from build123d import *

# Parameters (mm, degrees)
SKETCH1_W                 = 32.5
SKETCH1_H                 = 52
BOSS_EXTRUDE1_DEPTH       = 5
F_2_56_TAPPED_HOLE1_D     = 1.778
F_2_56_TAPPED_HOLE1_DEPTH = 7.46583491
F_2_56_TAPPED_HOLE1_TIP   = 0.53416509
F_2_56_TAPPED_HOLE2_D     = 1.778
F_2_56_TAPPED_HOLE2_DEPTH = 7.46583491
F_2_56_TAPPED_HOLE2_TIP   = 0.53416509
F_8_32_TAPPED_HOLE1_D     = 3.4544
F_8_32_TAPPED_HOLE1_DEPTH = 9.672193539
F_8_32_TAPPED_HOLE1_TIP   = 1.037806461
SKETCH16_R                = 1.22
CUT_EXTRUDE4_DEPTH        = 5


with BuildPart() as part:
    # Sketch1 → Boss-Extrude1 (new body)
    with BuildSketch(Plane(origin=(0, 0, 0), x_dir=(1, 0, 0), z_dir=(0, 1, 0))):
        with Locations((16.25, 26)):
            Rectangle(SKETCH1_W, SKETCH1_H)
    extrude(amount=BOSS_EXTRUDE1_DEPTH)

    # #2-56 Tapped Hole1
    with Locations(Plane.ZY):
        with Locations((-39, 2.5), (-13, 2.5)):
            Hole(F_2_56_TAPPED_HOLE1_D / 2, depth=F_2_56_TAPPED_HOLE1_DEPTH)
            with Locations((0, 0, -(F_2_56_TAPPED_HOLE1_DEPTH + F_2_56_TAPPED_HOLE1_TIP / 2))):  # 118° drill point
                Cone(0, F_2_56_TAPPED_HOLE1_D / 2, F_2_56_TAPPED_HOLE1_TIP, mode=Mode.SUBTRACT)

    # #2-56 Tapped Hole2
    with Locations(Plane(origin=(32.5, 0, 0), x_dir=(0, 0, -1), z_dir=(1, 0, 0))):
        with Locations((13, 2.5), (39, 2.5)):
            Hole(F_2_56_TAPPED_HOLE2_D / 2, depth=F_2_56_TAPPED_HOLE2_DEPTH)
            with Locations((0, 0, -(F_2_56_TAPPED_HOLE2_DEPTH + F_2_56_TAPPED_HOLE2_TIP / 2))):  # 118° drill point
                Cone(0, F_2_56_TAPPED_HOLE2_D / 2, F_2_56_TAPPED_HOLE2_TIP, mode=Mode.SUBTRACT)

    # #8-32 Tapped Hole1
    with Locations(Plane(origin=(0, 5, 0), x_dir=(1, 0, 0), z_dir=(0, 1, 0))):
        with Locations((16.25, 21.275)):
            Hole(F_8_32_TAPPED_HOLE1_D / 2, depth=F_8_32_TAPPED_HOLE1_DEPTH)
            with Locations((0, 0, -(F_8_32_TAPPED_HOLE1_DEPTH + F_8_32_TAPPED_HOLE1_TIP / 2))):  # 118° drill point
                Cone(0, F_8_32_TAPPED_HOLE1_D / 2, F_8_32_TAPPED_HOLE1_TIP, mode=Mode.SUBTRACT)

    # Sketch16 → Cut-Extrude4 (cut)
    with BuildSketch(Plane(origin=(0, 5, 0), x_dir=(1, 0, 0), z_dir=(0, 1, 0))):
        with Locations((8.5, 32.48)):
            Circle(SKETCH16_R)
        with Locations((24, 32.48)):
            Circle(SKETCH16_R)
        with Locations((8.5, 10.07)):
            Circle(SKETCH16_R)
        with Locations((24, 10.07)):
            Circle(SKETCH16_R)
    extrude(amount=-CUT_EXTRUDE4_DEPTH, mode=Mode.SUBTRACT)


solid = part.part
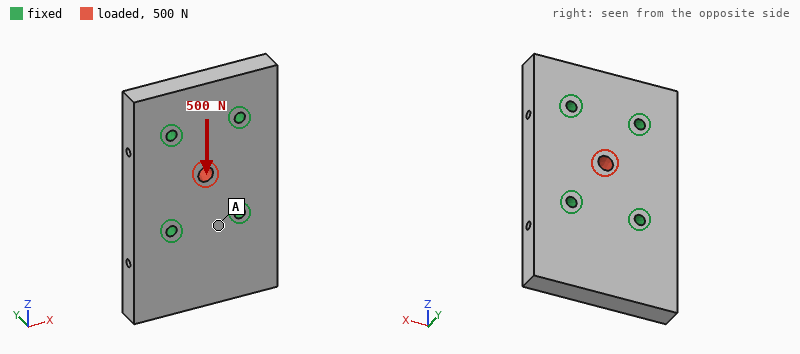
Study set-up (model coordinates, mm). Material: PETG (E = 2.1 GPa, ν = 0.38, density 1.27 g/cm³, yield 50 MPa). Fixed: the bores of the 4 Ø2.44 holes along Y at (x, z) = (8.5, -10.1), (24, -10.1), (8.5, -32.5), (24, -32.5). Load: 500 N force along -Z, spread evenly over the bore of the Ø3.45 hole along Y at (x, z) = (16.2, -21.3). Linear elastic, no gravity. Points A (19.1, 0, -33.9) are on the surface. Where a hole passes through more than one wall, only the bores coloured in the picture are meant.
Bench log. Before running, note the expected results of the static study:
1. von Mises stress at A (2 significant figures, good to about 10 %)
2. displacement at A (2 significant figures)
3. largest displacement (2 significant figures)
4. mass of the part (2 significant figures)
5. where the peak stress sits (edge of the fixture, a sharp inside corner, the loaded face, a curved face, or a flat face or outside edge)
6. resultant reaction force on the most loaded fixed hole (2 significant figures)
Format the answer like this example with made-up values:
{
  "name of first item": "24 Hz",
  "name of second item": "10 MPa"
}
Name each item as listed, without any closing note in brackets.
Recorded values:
{
  "von Mises stress at A": "1.5 MPa",
  "displacement at A": "7.1 µm",
  "largest displacement": "30 µm",
  "mass of the part": "10 g",
  "where the peak stress sits": "the loaded face",
  "resultant reaction force on the most loaded fixed hole": "130 N"
}
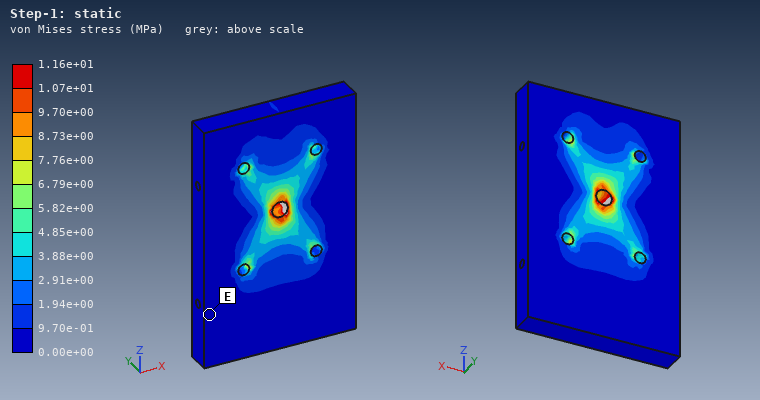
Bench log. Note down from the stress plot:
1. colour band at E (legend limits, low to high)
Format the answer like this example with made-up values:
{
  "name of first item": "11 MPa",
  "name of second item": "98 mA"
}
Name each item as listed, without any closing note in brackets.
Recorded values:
{
  "colour band at E": "0.00e+00 to 9.70e-01 MPa"
}
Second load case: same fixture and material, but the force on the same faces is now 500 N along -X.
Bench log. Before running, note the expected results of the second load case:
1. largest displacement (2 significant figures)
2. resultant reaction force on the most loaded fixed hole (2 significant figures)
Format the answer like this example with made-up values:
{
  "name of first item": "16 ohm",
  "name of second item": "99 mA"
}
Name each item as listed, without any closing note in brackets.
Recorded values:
{
  "largest displacement": "39 µm",
  "resultant reaction force on the most loaded fixed hole": "140 N"
}
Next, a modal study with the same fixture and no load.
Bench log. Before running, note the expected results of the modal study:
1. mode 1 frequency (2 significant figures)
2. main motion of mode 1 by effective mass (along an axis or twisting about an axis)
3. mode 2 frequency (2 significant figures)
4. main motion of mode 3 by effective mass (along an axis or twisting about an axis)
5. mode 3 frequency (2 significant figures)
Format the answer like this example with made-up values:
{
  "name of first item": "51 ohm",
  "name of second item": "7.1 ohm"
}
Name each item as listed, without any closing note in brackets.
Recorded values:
{
  "mode 1 frequency": "2400 Hz",
  "main motion of mode 1 by effective mass": "along Y",
  "mode 2 frequency": "3700 Hz",
  "main motion of mode 3 by effective mass": "along X",
  "mode 3 frequency": "6500 Hz"
}
